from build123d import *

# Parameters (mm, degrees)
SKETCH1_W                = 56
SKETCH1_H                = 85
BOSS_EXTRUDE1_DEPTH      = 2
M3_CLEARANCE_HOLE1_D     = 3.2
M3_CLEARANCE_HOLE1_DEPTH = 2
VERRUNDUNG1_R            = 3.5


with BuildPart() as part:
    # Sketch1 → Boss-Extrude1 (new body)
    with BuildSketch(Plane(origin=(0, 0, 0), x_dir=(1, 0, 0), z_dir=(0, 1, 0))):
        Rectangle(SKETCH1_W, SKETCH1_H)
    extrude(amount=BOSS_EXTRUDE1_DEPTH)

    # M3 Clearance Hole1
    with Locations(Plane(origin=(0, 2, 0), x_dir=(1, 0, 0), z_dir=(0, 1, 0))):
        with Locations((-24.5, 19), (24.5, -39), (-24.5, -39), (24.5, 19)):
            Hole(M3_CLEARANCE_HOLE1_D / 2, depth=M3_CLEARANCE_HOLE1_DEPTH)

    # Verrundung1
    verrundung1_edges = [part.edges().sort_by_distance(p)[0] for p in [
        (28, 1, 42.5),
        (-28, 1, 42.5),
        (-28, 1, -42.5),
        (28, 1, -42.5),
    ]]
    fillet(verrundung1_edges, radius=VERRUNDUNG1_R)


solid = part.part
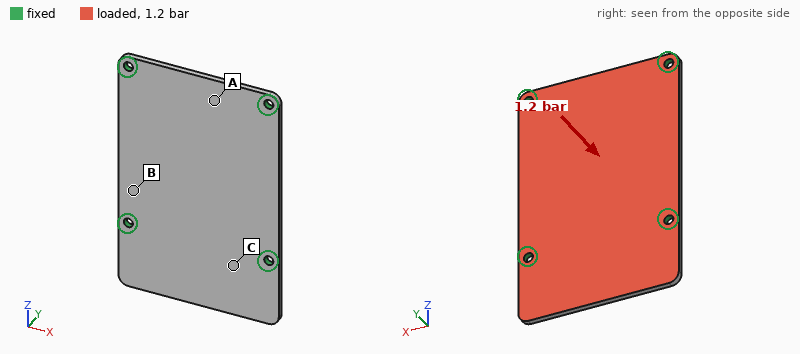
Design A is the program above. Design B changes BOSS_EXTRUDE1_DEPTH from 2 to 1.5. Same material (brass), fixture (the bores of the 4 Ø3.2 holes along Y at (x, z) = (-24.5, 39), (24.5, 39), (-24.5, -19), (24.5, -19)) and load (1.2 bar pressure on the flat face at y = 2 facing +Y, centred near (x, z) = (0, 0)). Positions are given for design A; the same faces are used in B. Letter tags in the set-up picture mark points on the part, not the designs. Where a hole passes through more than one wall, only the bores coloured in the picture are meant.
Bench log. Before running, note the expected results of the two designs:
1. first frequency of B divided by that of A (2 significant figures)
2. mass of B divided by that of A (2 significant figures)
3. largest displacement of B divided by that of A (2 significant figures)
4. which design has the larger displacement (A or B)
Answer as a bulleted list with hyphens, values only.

- 0.76
- 0.75
- 2.3
- B
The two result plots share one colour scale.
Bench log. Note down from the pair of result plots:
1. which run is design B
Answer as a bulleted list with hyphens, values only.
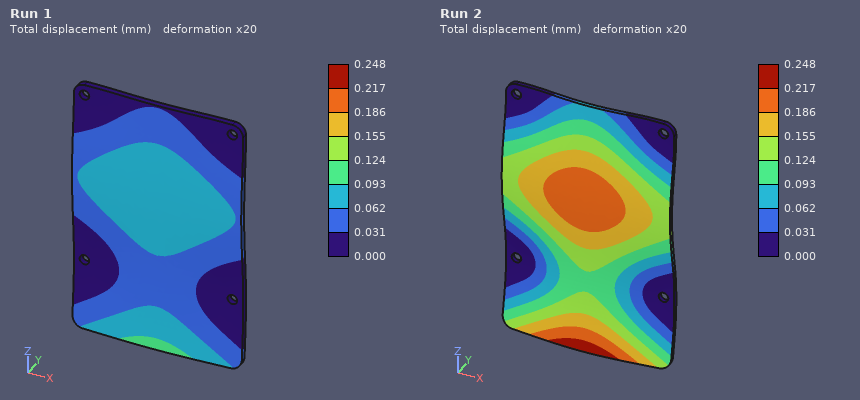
- Run 2
